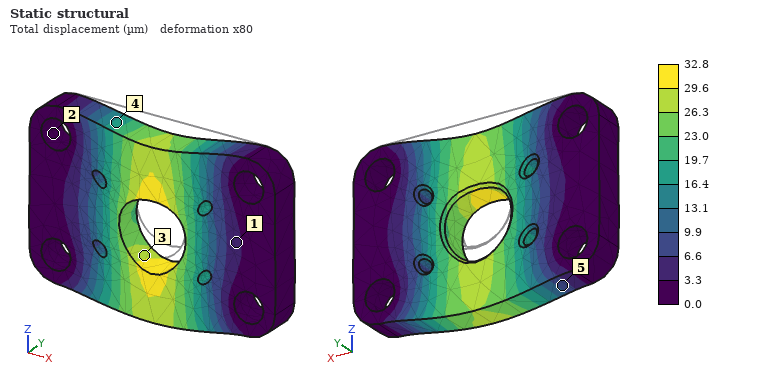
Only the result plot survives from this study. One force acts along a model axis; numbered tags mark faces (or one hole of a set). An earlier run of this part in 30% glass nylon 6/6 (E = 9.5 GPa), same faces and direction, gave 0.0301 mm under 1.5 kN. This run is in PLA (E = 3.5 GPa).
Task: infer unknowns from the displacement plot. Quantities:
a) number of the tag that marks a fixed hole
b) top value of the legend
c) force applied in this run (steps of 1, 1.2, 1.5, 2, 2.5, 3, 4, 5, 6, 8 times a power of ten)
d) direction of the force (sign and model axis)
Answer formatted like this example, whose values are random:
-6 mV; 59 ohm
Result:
2; 32.8 µm; 600 N; -Z
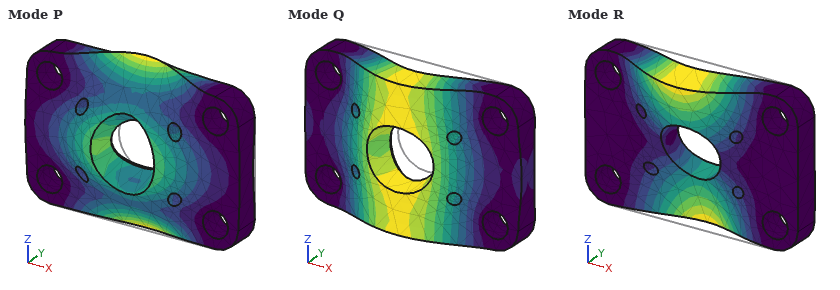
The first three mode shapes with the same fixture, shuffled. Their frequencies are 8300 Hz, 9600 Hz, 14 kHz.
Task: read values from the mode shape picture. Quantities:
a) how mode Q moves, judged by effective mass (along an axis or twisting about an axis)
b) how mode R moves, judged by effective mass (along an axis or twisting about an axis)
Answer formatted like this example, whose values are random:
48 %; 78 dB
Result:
along Y; twisting about X
